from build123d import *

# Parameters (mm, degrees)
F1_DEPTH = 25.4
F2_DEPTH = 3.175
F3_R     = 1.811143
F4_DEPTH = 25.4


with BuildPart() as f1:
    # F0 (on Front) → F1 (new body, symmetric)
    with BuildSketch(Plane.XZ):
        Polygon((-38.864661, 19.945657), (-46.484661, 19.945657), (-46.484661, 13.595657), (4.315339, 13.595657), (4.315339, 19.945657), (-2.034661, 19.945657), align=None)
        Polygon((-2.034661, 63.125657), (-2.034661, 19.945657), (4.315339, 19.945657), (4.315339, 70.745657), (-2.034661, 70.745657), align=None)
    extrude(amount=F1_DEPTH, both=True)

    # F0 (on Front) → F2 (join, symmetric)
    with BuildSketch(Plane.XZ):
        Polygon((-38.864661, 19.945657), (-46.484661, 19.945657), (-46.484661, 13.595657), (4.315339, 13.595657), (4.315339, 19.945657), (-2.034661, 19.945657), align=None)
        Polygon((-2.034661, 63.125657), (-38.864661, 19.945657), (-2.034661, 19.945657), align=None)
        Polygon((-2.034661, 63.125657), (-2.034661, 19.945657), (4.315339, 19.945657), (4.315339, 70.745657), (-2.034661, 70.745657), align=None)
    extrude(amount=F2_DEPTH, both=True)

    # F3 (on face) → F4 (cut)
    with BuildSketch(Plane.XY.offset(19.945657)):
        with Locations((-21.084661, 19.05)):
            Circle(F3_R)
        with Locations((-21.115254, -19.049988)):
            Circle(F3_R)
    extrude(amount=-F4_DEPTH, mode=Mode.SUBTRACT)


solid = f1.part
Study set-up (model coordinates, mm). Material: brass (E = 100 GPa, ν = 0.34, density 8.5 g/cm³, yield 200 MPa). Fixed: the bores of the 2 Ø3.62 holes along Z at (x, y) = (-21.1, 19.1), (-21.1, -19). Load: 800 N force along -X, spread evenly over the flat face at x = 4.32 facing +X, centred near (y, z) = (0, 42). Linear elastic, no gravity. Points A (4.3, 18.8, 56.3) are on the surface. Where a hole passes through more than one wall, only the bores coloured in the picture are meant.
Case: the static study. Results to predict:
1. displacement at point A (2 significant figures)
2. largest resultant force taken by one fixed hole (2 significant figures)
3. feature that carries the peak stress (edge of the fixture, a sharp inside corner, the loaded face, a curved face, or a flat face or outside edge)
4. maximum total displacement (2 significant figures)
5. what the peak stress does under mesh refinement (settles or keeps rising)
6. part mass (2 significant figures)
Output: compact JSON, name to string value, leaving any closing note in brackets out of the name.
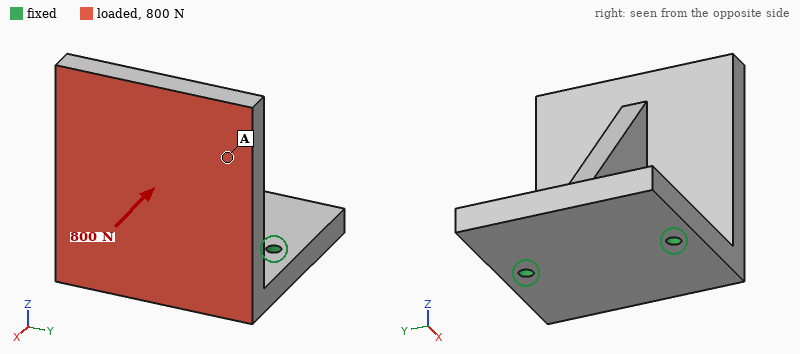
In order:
{"displacement at point A": "76 µm", "largest resultant force taken by one fixed hole": "400 N", "feature that carries the peak stress": "edge of the fixture", "maximum total displacement": "100 µm", "what the peak stress does under mesh refinement": "keeps rising", "part mass": "320 g"}
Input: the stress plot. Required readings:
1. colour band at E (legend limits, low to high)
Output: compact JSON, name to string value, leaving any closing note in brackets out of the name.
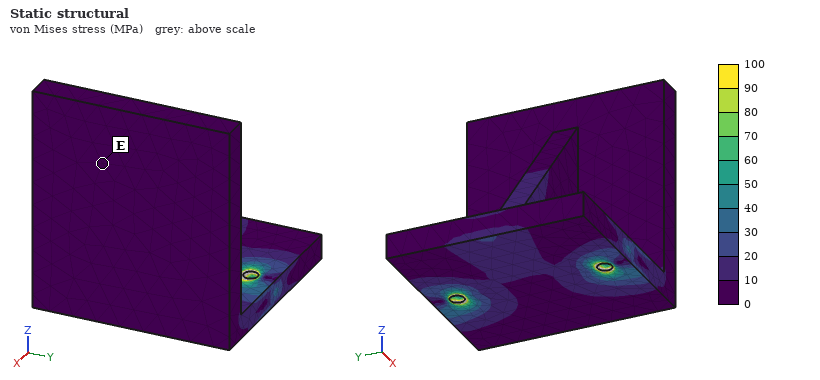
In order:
{"colour band at E": "0 to 10 MPa"}
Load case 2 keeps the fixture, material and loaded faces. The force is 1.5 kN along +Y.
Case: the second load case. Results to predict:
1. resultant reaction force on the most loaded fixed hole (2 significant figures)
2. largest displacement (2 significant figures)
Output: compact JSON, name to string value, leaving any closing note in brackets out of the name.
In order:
{"resultant reaction force on the most loaded fixed hole": "1.6 kN", "largest displacement": "92 µm"}
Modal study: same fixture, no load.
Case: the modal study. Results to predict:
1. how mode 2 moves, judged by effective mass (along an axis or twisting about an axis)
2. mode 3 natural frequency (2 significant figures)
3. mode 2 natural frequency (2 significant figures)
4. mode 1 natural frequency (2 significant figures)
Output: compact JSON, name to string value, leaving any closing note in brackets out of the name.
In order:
{"how mode 2 moves, judged by effective mass": "along Y", "mode 3 natural frequency": "3200 Hz", "mode 2 natural frequency": "1800 Hz", "mode 1 natural frequency": "1100 Hz"}
